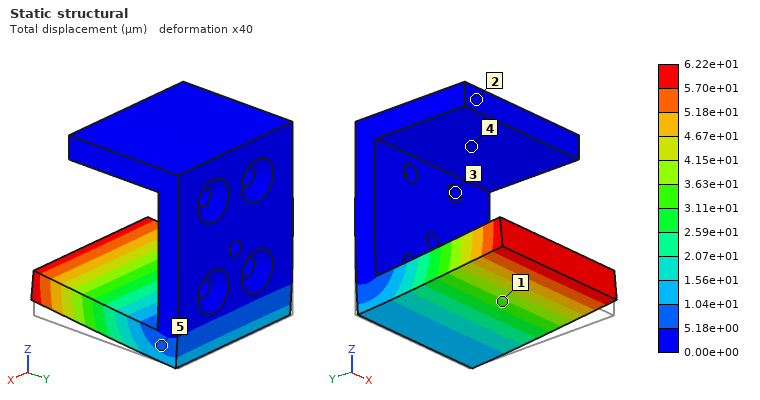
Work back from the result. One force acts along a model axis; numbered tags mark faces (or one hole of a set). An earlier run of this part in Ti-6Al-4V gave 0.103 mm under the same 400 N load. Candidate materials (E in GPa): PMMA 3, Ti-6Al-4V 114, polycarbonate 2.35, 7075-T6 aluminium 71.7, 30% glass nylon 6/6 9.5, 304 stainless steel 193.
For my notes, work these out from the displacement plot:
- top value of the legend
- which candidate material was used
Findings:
6.22e+01 µm
304 stainless steel
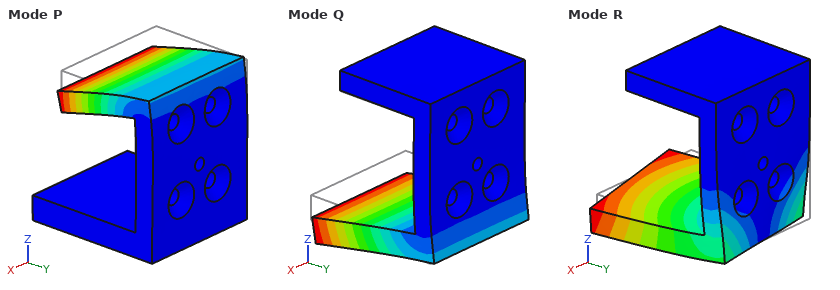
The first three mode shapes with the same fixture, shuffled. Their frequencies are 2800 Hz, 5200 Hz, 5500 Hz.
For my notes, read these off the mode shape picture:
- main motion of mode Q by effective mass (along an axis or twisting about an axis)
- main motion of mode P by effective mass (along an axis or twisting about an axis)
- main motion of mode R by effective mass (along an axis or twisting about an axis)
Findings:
along Z
along Z
along X
